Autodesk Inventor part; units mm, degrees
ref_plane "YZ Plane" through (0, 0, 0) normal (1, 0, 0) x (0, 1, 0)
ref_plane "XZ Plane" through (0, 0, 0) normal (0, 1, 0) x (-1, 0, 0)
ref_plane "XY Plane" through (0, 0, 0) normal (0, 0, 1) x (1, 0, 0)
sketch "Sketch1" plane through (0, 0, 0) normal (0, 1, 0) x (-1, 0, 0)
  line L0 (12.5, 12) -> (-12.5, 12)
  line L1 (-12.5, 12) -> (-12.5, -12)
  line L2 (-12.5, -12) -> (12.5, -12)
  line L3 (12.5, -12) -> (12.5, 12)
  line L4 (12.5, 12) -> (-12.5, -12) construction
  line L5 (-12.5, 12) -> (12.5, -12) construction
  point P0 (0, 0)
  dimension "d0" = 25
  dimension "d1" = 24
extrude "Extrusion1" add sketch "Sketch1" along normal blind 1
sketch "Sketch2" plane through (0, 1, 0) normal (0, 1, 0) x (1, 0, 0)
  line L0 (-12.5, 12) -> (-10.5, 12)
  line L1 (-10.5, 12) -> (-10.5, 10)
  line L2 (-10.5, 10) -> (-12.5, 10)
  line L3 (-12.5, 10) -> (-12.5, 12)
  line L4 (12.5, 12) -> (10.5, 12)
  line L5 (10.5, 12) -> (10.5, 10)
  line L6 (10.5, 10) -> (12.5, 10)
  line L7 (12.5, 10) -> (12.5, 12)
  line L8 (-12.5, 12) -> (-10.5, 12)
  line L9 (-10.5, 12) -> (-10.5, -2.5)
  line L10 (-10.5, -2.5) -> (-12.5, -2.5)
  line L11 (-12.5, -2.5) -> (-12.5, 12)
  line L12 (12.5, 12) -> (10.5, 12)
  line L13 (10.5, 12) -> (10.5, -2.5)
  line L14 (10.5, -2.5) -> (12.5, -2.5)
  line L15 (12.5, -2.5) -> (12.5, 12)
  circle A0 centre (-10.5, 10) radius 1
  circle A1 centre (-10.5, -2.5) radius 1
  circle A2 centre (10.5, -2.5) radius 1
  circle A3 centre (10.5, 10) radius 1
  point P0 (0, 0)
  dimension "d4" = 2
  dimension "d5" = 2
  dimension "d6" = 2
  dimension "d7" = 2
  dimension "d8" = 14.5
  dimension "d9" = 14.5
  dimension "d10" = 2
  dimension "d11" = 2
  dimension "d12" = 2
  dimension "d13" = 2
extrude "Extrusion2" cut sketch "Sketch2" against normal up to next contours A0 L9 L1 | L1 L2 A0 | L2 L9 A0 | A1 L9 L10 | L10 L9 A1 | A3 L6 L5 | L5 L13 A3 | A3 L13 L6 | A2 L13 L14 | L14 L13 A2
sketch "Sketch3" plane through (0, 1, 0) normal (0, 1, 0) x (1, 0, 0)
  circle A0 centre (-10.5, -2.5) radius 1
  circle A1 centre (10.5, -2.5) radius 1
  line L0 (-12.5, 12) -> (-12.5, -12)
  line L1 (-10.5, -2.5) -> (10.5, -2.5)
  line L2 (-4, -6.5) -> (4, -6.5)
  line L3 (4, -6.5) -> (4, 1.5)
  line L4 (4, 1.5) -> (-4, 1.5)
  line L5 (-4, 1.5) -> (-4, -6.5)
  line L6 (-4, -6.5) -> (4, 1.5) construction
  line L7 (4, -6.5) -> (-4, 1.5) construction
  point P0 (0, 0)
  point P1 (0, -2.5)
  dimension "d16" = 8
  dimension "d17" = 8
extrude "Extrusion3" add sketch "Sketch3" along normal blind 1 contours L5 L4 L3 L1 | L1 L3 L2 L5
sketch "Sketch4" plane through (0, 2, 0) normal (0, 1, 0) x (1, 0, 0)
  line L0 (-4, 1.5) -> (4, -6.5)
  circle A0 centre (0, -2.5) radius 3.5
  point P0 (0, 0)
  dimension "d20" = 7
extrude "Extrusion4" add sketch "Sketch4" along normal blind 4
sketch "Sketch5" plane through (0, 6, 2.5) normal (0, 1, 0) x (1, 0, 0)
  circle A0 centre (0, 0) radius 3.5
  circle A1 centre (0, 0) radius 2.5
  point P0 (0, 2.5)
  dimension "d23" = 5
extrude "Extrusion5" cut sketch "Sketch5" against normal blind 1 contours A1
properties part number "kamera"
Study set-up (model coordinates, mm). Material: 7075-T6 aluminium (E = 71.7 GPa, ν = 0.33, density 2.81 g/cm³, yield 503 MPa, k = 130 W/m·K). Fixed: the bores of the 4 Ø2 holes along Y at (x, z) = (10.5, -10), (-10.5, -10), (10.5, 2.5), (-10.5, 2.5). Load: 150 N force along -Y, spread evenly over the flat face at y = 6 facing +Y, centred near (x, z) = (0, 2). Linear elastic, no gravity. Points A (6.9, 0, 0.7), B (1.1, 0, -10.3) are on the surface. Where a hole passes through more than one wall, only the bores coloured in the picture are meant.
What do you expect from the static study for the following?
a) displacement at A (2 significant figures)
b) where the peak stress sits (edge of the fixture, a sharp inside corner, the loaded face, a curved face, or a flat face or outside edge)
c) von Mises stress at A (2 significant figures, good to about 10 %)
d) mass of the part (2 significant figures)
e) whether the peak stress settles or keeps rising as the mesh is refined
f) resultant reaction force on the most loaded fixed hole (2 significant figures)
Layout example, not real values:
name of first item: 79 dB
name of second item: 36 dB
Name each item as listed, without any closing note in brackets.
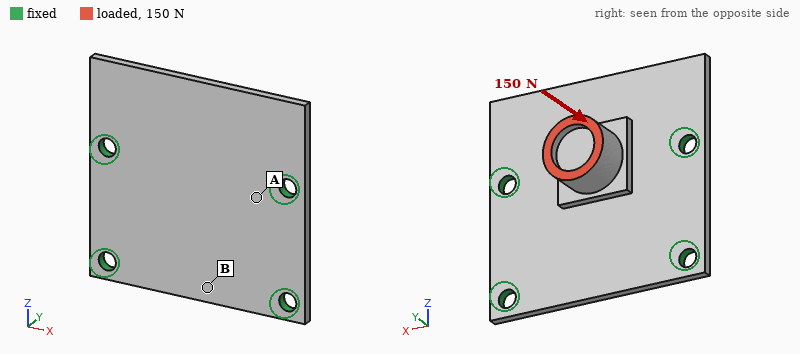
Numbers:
displacement at A: 15 µm
where the peak stress sits: edge of the fixture
von Mises stress at A: 36 MPa
mass of the part: 2.2 g
whether the peak stress settles or keeps rising as the mesh is refined: keeps rising
resultant reaction force on the most loaded fixed hole: 78 N
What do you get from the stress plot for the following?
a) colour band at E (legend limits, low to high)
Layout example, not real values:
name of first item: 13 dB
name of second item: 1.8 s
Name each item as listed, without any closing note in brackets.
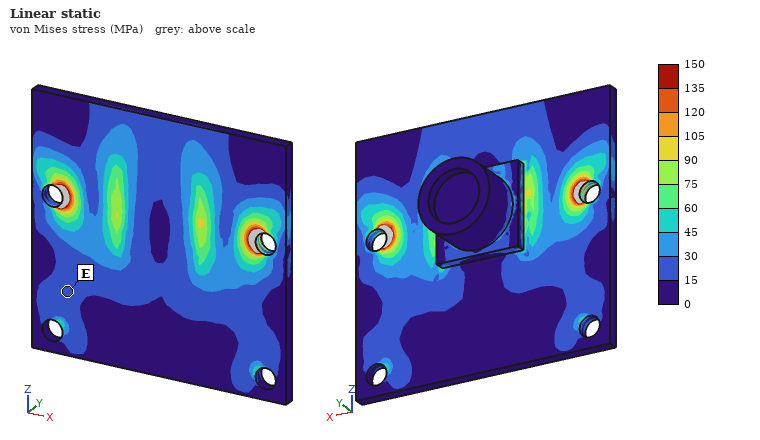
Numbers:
colour band at E: 15 to 30 MPa
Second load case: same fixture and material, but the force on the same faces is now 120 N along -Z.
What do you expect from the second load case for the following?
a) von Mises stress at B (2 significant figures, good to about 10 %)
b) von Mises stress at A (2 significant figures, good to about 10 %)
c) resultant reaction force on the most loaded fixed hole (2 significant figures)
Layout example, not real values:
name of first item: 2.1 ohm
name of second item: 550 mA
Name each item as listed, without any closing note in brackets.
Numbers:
von Mises stress at B: 29 MPa
von Mises stress at A: 52 MPa
resultant reaction force on the most loaded fixed hole: 41 N
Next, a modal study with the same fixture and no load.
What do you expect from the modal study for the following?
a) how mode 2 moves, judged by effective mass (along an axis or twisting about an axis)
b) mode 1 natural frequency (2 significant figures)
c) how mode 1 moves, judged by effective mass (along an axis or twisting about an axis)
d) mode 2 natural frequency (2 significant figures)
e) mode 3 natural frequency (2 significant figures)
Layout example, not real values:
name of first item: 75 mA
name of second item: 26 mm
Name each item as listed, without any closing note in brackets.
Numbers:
how mode 2 moves, judged by effective mass: along Y
mode 1 natural frequency: 7700 Hz
how mode 1 moves, judged by effective mass: along Y
mode 2 natural frequency: 11 kHz
mode 3 natural frequency: 14 kHz
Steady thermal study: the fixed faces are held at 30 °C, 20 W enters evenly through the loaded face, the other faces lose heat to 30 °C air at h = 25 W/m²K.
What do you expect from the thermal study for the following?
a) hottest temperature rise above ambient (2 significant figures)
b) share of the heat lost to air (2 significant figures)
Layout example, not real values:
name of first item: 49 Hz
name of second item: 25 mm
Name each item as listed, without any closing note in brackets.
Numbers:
hottest temperature rise above ambient: 69 K
share of the heat lost to air: 4.0 %
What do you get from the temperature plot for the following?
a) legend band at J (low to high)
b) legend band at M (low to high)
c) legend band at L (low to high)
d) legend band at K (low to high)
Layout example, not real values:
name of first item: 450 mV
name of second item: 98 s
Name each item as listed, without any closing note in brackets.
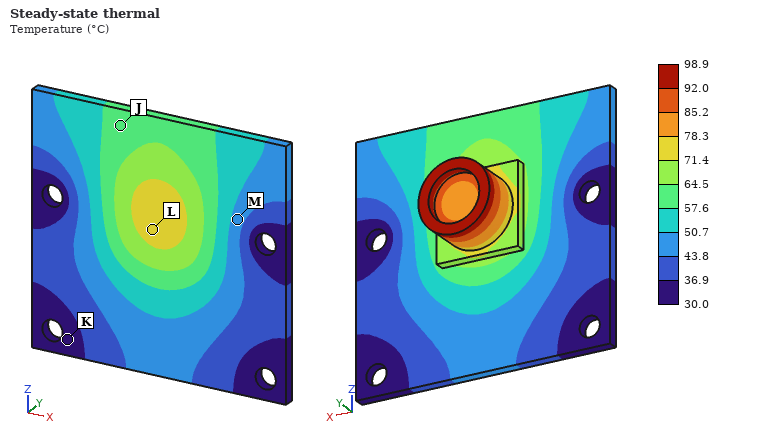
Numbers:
legend band at J: 57.6 to 64.5 °C
legend band at M: 43.8 to 50.7 °C
legend band at L: 71.4 to 78.3 °C
legend band at K: 30.0 to 36.9 °C
